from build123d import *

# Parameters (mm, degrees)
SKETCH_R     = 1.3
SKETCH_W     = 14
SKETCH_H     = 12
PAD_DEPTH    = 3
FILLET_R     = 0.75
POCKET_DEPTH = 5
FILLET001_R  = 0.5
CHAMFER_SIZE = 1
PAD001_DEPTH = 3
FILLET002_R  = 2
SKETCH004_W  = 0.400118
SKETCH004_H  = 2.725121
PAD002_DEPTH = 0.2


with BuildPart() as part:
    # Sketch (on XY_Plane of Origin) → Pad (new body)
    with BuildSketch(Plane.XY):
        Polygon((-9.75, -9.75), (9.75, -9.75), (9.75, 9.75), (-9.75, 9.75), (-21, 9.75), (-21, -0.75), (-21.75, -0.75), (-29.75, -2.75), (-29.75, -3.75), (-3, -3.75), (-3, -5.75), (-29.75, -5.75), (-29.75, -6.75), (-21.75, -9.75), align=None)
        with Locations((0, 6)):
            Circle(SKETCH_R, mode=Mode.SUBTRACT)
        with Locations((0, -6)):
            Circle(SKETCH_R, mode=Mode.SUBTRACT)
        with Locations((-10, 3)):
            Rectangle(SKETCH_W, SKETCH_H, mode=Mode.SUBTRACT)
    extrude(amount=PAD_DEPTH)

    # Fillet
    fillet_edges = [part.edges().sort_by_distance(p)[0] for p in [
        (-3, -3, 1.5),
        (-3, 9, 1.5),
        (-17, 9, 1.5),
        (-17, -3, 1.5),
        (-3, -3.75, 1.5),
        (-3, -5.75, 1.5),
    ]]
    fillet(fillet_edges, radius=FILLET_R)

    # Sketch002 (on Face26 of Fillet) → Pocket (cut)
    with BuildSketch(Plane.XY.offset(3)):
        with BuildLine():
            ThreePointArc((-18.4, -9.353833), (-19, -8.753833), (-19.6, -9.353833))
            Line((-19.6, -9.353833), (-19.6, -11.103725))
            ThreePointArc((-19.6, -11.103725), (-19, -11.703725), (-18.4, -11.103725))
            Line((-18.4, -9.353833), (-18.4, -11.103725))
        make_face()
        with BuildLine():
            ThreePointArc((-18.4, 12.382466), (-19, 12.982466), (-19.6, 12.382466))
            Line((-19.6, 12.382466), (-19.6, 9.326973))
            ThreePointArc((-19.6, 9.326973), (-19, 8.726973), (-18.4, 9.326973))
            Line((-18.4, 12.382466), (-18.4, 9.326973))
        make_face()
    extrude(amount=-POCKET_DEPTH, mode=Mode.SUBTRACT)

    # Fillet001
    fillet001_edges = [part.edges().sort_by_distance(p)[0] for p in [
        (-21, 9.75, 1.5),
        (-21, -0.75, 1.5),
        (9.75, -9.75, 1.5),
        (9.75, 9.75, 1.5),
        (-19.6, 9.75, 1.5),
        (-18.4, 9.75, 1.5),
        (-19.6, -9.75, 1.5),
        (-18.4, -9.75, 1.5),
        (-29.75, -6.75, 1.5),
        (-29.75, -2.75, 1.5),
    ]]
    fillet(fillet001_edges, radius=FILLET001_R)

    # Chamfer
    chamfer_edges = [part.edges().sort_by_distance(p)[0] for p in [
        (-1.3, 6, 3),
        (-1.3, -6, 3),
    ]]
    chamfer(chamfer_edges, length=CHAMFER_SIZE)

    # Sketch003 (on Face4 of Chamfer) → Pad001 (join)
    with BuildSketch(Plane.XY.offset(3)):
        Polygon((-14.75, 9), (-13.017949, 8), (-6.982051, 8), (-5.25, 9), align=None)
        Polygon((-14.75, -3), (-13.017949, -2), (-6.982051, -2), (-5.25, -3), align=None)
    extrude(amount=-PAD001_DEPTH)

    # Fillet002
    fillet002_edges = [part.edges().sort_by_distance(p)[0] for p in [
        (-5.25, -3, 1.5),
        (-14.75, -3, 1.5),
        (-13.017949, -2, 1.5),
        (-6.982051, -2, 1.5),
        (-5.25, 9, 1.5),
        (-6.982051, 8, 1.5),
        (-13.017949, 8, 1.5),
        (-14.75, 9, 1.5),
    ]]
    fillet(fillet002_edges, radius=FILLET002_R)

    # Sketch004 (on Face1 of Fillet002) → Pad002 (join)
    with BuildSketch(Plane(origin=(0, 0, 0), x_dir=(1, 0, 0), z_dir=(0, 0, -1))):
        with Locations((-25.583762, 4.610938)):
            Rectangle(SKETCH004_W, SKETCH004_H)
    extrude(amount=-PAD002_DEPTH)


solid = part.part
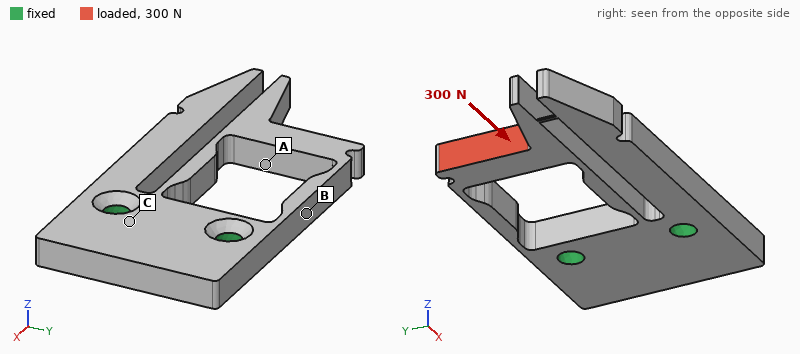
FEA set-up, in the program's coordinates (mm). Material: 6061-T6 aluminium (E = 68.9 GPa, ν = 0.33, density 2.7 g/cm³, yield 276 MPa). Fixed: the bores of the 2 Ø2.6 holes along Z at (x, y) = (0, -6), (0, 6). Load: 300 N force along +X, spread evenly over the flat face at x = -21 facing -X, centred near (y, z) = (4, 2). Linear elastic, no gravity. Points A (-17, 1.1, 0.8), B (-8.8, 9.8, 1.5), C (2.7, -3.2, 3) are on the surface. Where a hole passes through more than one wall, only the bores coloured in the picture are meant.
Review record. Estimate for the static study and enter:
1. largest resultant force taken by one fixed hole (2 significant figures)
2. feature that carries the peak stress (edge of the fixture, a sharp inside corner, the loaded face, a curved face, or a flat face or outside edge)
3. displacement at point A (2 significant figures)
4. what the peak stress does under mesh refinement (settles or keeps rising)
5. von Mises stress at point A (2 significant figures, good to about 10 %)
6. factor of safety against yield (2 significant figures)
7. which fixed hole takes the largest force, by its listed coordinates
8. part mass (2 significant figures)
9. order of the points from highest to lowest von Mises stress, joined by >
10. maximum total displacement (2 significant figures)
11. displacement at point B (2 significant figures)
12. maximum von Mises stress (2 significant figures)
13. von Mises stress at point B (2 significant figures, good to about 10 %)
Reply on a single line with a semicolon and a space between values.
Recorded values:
230 N; a curved face; 25 µm; settles; 58 MPa; 1.5; (0, 6); 3.5 g; B > A > C; 27 µm; 12 µm; 190 MPa; 80 MPa
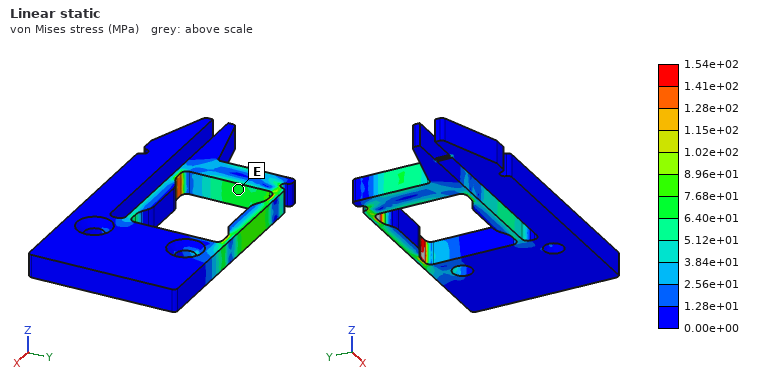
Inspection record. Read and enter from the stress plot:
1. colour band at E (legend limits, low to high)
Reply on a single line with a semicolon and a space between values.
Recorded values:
6.40e+01 to 7.68e+01 MPa
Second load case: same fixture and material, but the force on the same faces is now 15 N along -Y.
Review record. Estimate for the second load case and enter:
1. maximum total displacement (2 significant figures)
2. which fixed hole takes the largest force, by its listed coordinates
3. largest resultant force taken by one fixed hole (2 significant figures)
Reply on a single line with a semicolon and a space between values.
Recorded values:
61 µm; (0, -6); 19 N
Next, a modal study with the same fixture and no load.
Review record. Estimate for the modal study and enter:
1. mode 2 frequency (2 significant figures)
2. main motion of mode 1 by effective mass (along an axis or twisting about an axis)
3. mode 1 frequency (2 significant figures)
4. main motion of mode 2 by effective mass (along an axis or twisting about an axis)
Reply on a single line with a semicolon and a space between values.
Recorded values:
2800 Hz; along Z; 2500 Hz; along Y
